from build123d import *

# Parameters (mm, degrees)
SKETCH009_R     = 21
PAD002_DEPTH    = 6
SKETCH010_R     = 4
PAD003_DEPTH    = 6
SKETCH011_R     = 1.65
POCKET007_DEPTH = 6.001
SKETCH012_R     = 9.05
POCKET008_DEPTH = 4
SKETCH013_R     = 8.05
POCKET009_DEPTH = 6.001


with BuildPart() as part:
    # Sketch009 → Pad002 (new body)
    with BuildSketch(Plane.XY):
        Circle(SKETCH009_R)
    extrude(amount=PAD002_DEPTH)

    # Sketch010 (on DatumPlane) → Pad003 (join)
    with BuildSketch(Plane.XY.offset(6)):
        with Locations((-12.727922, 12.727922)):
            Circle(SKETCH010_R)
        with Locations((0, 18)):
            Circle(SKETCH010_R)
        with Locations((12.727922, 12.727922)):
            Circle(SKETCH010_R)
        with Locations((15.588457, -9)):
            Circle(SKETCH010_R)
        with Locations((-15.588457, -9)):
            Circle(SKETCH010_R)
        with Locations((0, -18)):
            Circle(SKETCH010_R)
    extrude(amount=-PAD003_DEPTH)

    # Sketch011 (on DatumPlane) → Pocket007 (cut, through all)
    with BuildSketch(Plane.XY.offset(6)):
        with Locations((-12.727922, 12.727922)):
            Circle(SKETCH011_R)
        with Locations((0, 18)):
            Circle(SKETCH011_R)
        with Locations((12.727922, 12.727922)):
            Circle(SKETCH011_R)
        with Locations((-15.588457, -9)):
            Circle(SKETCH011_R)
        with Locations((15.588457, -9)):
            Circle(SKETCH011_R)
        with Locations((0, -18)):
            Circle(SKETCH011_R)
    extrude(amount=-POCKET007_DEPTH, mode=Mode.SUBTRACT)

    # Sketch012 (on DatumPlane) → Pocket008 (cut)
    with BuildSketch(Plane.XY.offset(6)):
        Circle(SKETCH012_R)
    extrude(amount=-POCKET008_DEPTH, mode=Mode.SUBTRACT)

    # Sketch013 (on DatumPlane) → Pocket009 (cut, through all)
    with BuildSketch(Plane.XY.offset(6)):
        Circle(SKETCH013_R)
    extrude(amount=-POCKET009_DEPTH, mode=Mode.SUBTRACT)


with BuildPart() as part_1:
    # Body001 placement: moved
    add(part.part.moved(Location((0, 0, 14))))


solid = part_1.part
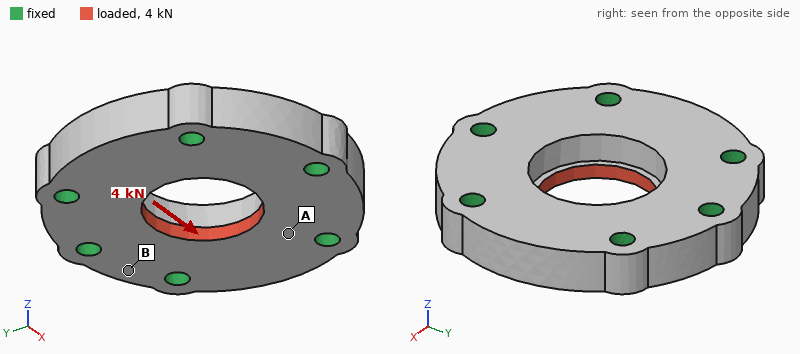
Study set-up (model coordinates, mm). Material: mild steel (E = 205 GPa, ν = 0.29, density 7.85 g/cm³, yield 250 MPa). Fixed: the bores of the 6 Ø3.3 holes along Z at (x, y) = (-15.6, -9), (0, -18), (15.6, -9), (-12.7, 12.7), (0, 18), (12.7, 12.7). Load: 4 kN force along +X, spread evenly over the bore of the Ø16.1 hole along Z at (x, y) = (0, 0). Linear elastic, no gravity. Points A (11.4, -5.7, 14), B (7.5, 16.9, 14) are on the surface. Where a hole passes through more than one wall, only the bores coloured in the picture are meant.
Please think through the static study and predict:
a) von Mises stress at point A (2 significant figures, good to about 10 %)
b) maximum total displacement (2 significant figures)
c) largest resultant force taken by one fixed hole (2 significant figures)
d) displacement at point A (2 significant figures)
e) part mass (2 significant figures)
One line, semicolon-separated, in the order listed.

36 MPa; 2.5 µm; 940 N; 0.79 µm; 53 g
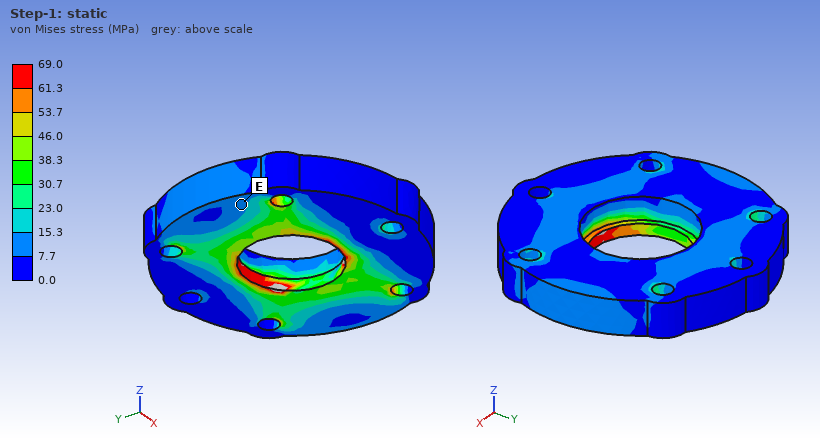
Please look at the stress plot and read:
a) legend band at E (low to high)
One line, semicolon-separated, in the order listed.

7.7 to 15.3 MPa
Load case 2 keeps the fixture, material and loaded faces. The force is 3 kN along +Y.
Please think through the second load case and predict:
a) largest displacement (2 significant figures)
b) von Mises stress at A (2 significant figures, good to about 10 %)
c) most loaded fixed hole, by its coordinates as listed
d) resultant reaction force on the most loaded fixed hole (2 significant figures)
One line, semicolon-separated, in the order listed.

1.5 µm; 13 MPa; (0, -18); 750 N
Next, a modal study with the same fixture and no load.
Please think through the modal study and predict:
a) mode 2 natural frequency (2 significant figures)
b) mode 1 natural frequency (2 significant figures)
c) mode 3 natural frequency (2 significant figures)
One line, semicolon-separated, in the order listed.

46 kHz; 44 kHz; 48 kHz
